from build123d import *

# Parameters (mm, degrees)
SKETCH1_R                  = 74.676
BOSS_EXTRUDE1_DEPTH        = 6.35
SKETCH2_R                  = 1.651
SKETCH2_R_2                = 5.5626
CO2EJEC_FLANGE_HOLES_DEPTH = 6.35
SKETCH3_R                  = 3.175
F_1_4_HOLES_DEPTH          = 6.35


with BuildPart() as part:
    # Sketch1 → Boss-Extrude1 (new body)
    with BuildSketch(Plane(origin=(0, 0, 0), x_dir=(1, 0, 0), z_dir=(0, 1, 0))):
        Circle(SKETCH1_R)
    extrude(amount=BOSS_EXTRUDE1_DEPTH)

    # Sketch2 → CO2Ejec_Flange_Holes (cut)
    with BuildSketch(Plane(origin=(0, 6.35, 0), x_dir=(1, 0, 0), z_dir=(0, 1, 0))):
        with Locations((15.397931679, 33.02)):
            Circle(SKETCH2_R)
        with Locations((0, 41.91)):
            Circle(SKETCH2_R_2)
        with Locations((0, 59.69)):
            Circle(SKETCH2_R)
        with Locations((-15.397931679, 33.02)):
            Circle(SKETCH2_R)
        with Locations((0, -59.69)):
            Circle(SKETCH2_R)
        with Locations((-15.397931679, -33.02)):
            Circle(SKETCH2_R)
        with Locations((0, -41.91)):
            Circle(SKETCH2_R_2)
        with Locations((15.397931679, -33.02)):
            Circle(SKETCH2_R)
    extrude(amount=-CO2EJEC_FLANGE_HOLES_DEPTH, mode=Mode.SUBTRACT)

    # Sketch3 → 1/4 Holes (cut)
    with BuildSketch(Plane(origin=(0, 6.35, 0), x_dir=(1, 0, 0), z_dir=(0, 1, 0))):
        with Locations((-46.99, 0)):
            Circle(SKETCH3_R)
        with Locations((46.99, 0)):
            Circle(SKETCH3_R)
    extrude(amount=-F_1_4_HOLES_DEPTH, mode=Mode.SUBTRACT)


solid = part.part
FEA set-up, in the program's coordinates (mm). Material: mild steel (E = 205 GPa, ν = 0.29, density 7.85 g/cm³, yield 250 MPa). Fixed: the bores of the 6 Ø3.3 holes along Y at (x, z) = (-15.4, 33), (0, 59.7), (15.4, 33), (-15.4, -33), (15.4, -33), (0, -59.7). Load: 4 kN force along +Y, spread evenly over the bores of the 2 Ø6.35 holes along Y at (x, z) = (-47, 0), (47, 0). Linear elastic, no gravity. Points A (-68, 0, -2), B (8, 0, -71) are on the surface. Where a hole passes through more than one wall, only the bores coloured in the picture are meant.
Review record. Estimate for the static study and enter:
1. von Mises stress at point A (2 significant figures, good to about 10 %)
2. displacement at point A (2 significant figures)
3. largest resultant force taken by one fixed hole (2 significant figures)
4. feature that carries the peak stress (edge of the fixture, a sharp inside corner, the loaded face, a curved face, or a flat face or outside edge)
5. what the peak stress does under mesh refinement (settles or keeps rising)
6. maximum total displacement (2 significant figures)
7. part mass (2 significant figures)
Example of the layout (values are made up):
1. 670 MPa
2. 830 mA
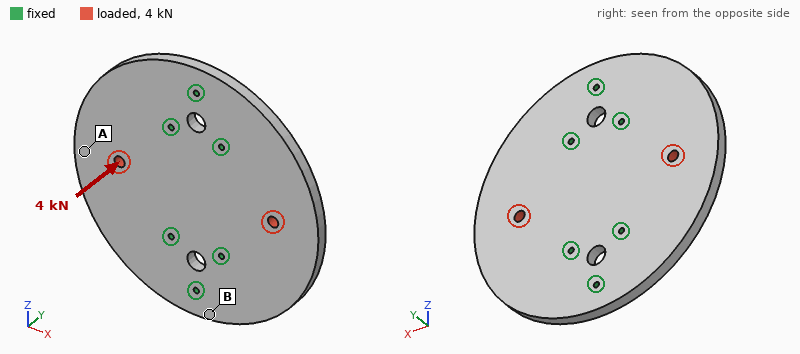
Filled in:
1. 41 MPa
2. 0.14 mm
3. 1.4 kN
4. edge of the fixture
5. keeps rising
6. 0.16 mm
7. 860 g
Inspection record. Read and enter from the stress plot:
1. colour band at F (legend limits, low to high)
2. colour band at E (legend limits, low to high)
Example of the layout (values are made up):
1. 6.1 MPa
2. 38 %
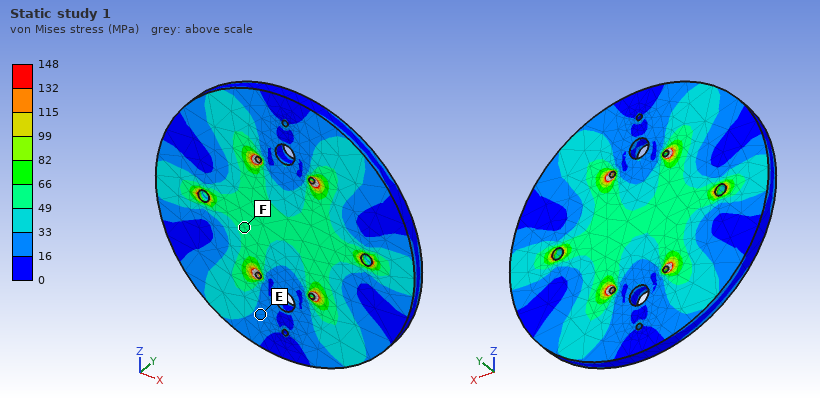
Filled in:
1. 49 to 66 MPa
2. 16 to 33 MPa
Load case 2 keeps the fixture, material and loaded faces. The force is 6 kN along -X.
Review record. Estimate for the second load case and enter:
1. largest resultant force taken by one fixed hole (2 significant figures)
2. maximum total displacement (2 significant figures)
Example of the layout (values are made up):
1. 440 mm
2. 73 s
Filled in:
1. 1.3 kN
2. 3.1 µm
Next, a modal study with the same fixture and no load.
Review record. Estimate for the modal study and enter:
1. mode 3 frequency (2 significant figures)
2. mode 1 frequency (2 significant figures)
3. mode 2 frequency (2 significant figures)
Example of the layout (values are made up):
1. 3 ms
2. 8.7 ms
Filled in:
1. 3000 Hz
2. 1600 Hz
3. 1600 Hz
